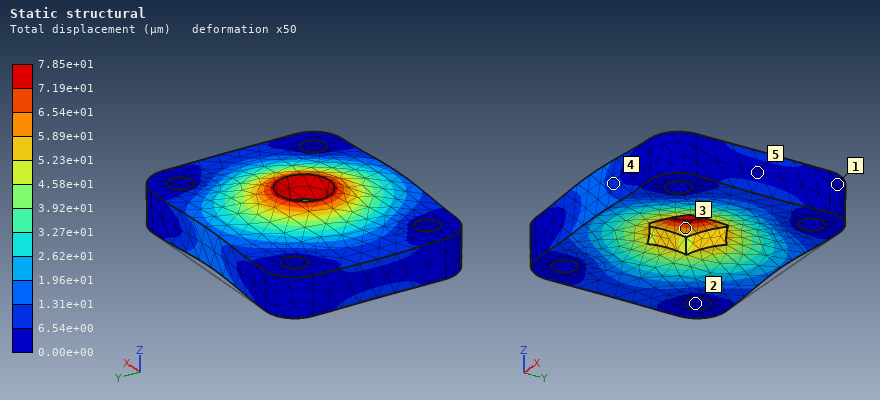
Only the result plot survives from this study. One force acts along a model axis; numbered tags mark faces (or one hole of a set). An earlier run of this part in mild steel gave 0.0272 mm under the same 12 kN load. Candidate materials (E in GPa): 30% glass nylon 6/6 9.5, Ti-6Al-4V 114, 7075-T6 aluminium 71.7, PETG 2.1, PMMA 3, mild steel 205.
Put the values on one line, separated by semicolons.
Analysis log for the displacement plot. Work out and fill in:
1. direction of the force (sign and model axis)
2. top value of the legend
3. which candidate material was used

+Z; 7.85e+01 µm; 7075-T6 aluminium
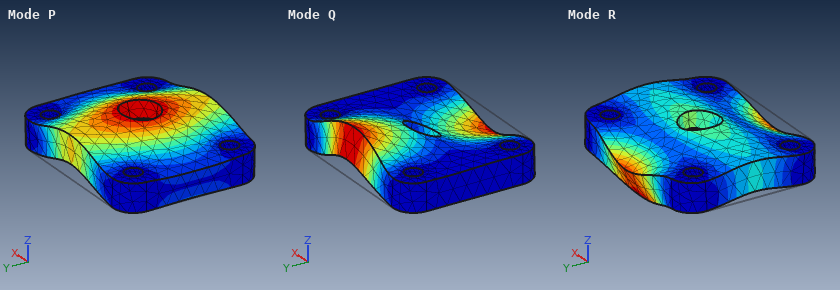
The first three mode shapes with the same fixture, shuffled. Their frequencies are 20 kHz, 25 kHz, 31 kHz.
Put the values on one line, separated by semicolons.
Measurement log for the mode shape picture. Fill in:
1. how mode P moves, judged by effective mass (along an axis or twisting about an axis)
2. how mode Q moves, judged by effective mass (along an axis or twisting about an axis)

along Z; twisting about X
